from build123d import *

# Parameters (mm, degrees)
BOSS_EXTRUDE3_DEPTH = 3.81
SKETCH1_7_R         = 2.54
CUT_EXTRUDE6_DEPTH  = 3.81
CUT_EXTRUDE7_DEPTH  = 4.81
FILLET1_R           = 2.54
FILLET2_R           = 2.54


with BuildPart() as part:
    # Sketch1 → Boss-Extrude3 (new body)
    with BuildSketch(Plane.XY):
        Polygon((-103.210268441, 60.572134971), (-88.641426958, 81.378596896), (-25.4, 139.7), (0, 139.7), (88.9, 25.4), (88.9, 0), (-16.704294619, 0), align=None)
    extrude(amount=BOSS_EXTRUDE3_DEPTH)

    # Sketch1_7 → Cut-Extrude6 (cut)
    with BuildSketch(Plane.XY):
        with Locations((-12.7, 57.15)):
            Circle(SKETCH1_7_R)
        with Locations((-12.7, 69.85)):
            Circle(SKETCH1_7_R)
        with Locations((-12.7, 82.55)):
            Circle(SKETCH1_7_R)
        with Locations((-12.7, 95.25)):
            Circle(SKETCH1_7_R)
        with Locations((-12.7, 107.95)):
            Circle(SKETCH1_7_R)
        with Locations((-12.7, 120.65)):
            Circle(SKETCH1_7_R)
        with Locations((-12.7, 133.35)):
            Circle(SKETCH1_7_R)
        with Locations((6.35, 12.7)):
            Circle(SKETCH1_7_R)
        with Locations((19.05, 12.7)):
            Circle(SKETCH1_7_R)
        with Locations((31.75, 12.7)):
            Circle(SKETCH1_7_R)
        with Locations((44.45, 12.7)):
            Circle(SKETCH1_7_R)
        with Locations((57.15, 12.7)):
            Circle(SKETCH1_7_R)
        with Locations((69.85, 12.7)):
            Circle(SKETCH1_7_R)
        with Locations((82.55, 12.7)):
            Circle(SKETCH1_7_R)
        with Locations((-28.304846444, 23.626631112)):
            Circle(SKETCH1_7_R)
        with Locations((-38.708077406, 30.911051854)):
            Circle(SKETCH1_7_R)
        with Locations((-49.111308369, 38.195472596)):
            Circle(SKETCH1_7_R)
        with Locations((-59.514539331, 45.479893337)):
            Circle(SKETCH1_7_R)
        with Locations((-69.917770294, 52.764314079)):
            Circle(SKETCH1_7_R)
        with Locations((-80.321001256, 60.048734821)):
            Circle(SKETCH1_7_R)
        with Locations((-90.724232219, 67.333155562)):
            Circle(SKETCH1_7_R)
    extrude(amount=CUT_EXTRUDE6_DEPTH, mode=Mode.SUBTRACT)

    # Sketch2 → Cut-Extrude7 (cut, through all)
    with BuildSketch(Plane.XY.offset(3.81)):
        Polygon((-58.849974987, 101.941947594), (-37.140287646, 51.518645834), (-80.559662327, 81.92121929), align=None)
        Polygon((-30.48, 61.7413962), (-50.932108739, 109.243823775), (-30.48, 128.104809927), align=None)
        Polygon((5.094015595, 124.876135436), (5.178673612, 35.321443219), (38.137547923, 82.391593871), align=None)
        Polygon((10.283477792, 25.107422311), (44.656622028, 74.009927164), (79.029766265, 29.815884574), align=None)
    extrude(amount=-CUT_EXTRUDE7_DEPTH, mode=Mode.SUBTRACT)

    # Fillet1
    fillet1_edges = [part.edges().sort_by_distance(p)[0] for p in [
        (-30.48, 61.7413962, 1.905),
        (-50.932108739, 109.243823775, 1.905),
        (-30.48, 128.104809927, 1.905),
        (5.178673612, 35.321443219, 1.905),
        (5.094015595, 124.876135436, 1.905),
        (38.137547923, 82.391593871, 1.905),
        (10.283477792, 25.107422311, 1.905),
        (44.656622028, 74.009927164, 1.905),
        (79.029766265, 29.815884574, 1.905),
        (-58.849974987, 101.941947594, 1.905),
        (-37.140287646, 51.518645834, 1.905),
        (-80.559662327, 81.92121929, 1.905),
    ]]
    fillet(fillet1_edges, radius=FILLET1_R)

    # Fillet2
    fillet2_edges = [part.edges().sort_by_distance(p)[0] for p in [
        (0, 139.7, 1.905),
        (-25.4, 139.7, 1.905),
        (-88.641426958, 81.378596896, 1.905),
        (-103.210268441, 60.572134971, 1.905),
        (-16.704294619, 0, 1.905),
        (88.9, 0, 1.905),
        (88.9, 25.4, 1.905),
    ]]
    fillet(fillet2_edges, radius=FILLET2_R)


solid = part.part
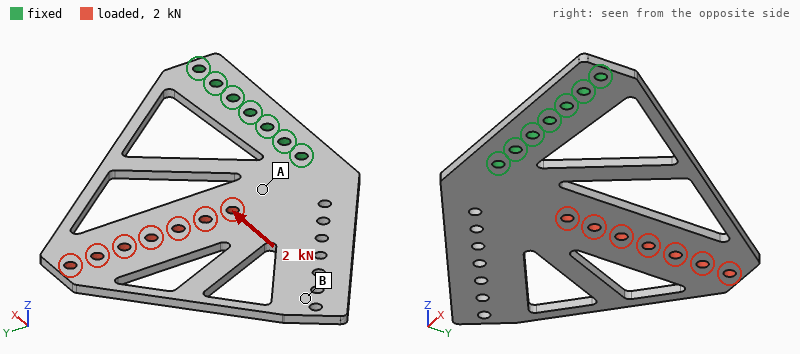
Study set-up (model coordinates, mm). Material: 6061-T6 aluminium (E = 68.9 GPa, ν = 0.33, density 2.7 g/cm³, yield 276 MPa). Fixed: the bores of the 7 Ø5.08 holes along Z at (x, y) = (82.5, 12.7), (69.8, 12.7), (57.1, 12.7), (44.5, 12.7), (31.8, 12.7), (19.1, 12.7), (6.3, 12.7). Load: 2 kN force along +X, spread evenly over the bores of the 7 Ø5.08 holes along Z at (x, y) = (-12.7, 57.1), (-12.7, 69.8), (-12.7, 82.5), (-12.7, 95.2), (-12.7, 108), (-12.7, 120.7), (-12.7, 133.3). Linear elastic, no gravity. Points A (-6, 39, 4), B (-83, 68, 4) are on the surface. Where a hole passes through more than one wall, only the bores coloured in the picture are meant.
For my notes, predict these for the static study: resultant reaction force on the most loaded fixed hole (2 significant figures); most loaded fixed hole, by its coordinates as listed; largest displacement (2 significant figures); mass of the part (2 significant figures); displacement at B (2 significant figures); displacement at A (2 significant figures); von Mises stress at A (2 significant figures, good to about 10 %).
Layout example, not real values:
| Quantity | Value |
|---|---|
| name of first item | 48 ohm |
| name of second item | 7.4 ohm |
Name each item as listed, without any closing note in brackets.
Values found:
| Quantity | Value |
|---|---|
| resultant reaction force on the most loaded fixed hole | 3.6 kN |
| most loaded fixed hole, by its coordinates as listed | (6.3, 12.7) |
| largest displacement | 0.33 mm |
| mass of the part | 120 g |
| displacement at B | 0.28 mm |
| displacement at A | 0.077 mm |
| von Mises stress at A | 25 MPa |
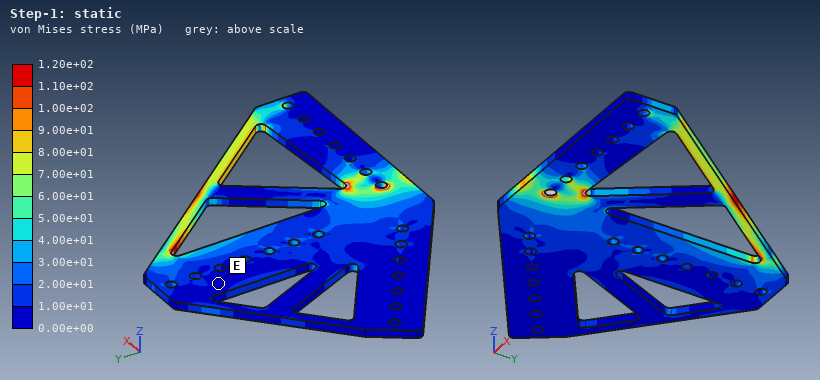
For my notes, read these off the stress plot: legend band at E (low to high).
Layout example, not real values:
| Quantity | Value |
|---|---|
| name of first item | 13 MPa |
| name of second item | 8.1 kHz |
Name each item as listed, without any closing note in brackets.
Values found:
| Quantity | Value |
|---|---|
| legend band at E | 0.00e+00 to 1.00e+01 MPa |
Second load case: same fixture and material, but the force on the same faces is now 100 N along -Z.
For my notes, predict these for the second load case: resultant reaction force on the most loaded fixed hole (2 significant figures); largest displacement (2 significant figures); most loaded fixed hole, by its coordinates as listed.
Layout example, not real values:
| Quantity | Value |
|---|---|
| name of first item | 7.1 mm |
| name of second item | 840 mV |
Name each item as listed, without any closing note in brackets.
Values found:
| Quantity | Value |
|---|---|
| resultant reaction force on the most loaded fixed hole | 160 N |
| largest displacement | 2.4 mm |
| most loaded fixed hole, by its coordinates as listed | (6.3, 12.7) |
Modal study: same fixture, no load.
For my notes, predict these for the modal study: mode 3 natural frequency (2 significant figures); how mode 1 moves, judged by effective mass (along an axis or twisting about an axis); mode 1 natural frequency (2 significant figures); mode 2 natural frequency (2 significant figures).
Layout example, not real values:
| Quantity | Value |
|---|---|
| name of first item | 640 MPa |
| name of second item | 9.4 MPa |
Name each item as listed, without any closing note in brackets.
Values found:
| Quantity | Value |
|---|---|
| mode 3 natural frequency | 950 Hz |
| how mode 1 moves, judged by effective mass | along Z |
| mode 1 natural frequency | 170 Hz |
| mode 2 natural frequency | 340 Hz |
